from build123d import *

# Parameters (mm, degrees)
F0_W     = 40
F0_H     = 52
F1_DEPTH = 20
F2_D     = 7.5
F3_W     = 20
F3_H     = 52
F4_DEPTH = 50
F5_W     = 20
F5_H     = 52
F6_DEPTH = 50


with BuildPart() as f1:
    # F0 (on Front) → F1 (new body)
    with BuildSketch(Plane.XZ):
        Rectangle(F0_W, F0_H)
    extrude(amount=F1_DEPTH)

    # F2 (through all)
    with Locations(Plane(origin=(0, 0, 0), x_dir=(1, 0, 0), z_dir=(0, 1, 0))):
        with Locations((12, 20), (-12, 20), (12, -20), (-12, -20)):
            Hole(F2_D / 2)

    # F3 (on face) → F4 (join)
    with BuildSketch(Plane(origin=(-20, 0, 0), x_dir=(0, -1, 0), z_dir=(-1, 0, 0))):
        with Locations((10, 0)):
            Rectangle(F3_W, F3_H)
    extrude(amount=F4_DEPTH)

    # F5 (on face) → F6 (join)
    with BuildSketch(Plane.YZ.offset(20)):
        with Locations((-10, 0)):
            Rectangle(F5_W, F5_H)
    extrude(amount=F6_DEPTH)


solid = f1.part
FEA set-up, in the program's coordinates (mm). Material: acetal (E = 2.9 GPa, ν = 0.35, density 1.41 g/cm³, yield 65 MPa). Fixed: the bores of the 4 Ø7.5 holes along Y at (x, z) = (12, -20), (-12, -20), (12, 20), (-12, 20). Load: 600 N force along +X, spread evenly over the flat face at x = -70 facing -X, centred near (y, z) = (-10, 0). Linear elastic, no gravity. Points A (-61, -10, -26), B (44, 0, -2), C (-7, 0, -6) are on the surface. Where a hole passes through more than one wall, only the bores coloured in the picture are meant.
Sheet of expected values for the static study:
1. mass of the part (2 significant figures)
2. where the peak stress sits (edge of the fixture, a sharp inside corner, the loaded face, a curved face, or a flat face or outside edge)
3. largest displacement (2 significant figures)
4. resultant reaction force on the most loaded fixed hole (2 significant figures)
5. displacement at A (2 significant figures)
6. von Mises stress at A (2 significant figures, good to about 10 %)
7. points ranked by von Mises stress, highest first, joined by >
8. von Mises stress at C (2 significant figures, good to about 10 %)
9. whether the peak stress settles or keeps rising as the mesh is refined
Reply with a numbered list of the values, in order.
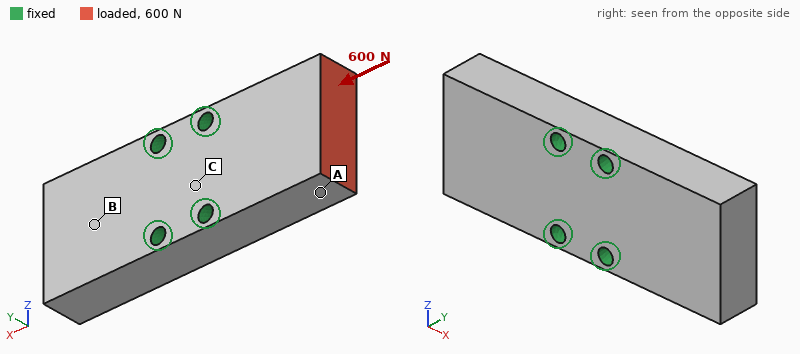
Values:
1. 200 g
2. edge of the fixture
3. 12 µm
4. 260 N
5. 10 µm
6. 0.57 MPa
7. A > C > B
8. 0.26 MPa
9. keeps rising
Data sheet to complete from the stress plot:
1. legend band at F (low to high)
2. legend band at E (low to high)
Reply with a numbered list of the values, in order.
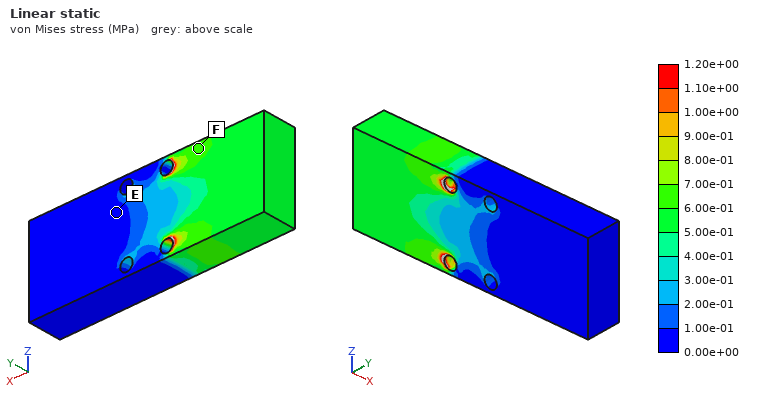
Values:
1. 6.00e-01 to 7.00e-01 MPa
2. 0.00e+00 to 1.00e-01 MPa
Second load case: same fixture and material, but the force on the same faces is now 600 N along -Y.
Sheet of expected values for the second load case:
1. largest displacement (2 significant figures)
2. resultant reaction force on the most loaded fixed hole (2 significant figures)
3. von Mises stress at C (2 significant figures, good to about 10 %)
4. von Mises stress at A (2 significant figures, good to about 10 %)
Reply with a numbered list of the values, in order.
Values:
1. 0.45 mm
2. 430 N
3. 3.5 MPa
4. 2.1 MPa
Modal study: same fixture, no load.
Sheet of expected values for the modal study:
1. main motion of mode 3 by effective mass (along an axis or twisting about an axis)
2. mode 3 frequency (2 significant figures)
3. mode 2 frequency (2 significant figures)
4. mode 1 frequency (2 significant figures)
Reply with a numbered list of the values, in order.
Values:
1. twisting about Y
2. 2500 Hz
3. 1200 Hz
4. 1200 Hz
